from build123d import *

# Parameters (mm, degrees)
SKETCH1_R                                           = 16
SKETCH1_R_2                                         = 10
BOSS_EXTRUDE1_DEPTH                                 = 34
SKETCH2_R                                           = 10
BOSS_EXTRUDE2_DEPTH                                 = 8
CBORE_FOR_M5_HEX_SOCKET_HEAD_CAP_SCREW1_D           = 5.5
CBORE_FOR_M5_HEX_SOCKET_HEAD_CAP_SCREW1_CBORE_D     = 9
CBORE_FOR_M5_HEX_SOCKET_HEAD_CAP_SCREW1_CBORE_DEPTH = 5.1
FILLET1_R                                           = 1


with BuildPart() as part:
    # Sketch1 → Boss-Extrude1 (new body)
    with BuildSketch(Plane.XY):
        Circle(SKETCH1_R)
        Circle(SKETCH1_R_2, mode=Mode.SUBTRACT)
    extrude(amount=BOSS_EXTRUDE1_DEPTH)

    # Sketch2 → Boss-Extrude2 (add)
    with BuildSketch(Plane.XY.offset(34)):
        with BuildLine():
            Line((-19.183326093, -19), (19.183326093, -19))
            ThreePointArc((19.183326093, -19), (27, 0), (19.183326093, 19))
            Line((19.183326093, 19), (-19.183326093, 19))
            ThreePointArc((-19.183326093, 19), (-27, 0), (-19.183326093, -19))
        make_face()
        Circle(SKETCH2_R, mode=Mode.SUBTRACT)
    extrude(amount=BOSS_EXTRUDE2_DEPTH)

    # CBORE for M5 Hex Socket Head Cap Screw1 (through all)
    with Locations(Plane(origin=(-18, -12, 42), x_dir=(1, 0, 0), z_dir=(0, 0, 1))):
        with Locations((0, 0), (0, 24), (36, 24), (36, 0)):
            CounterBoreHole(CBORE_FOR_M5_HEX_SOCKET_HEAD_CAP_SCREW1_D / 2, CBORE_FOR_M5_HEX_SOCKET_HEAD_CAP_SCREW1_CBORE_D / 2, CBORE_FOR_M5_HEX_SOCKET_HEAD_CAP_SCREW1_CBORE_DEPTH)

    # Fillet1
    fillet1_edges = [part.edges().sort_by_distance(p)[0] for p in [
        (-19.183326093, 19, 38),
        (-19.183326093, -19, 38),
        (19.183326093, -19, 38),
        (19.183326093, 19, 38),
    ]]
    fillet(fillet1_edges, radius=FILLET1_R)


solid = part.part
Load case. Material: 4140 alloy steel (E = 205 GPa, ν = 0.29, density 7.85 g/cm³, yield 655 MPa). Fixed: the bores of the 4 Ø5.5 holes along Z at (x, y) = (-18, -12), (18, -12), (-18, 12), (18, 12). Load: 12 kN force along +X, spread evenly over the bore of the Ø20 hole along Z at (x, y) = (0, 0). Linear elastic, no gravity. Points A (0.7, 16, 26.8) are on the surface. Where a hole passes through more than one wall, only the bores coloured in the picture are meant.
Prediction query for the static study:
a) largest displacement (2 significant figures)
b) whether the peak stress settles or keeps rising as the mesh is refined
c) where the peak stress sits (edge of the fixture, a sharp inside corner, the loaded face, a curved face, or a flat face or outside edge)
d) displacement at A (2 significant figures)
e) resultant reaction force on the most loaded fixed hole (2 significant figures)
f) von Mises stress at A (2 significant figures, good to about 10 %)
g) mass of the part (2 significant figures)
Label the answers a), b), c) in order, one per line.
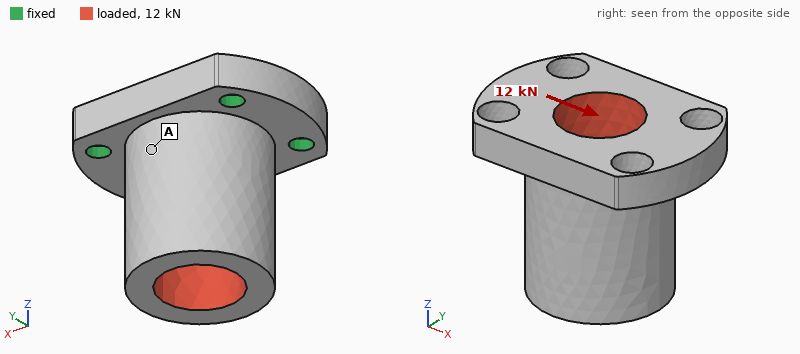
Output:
a) 31 µm
b) keeps rising
c) edge of the fixture
d) 8.6 µm
e) 4.0 kN
f) 29 MPa
g) 220 g
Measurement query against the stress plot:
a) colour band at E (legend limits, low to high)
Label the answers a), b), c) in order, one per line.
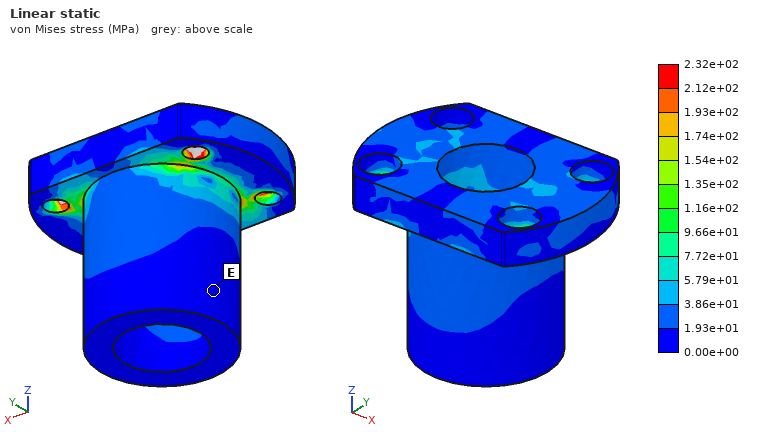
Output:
a) 0.00e+00 to 1.93e+01 MPa
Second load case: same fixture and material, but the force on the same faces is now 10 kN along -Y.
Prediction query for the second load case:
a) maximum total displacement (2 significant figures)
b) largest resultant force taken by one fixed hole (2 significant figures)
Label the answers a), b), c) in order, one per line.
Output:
a) 43 µm
b) 3.9 kN
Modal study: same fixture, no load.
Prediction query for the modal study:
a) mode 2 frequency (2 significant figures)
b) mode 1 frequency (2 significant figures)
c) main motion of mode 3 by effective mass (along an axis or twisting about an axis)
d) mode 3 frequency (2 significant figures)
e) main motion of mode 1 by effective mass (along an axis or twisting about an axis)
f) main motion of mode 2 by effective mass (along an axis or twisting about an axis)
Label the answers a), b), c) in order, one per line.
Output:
a) 9100 Hz
b) 7000 Hz
c) along Z
d) 14 kHz
e) along Y
f) along X
